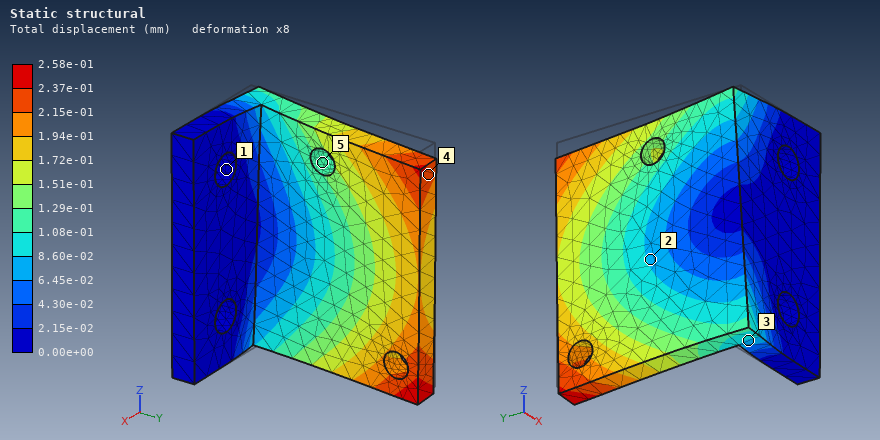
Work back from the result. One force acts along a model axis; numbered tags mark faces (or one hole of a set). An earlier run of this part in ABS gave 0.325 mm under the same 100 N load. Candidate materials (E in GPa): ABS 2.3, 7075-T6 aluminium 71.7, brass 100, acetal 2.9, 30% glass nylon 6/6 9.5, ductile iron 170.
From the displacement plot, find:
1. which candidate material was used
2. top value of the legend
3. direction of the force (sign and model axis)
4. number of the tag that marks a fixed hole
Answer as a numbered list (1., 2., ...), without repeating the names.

1. acetal
2. 2.58e-01 mm
3. -Z
4. 1
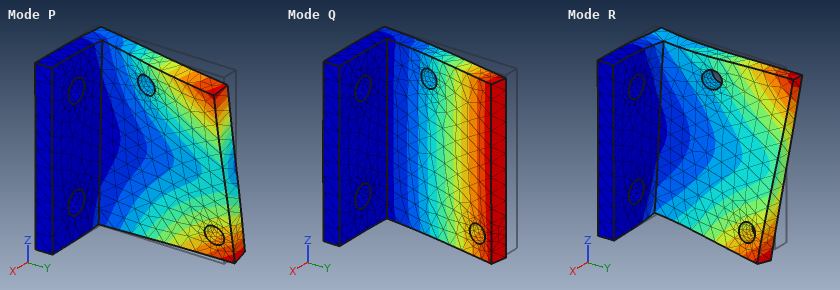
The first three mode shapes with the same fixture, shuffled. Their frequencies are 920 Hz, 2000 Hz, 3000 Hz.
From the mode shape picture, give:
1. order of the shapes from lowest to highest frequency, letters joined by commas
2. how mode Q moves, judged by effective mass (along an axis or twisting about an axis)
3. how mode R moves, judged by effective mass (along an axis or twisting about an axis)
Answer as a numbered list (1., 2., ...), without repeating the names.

1. Q, P, R
2. along X
3. along Z
